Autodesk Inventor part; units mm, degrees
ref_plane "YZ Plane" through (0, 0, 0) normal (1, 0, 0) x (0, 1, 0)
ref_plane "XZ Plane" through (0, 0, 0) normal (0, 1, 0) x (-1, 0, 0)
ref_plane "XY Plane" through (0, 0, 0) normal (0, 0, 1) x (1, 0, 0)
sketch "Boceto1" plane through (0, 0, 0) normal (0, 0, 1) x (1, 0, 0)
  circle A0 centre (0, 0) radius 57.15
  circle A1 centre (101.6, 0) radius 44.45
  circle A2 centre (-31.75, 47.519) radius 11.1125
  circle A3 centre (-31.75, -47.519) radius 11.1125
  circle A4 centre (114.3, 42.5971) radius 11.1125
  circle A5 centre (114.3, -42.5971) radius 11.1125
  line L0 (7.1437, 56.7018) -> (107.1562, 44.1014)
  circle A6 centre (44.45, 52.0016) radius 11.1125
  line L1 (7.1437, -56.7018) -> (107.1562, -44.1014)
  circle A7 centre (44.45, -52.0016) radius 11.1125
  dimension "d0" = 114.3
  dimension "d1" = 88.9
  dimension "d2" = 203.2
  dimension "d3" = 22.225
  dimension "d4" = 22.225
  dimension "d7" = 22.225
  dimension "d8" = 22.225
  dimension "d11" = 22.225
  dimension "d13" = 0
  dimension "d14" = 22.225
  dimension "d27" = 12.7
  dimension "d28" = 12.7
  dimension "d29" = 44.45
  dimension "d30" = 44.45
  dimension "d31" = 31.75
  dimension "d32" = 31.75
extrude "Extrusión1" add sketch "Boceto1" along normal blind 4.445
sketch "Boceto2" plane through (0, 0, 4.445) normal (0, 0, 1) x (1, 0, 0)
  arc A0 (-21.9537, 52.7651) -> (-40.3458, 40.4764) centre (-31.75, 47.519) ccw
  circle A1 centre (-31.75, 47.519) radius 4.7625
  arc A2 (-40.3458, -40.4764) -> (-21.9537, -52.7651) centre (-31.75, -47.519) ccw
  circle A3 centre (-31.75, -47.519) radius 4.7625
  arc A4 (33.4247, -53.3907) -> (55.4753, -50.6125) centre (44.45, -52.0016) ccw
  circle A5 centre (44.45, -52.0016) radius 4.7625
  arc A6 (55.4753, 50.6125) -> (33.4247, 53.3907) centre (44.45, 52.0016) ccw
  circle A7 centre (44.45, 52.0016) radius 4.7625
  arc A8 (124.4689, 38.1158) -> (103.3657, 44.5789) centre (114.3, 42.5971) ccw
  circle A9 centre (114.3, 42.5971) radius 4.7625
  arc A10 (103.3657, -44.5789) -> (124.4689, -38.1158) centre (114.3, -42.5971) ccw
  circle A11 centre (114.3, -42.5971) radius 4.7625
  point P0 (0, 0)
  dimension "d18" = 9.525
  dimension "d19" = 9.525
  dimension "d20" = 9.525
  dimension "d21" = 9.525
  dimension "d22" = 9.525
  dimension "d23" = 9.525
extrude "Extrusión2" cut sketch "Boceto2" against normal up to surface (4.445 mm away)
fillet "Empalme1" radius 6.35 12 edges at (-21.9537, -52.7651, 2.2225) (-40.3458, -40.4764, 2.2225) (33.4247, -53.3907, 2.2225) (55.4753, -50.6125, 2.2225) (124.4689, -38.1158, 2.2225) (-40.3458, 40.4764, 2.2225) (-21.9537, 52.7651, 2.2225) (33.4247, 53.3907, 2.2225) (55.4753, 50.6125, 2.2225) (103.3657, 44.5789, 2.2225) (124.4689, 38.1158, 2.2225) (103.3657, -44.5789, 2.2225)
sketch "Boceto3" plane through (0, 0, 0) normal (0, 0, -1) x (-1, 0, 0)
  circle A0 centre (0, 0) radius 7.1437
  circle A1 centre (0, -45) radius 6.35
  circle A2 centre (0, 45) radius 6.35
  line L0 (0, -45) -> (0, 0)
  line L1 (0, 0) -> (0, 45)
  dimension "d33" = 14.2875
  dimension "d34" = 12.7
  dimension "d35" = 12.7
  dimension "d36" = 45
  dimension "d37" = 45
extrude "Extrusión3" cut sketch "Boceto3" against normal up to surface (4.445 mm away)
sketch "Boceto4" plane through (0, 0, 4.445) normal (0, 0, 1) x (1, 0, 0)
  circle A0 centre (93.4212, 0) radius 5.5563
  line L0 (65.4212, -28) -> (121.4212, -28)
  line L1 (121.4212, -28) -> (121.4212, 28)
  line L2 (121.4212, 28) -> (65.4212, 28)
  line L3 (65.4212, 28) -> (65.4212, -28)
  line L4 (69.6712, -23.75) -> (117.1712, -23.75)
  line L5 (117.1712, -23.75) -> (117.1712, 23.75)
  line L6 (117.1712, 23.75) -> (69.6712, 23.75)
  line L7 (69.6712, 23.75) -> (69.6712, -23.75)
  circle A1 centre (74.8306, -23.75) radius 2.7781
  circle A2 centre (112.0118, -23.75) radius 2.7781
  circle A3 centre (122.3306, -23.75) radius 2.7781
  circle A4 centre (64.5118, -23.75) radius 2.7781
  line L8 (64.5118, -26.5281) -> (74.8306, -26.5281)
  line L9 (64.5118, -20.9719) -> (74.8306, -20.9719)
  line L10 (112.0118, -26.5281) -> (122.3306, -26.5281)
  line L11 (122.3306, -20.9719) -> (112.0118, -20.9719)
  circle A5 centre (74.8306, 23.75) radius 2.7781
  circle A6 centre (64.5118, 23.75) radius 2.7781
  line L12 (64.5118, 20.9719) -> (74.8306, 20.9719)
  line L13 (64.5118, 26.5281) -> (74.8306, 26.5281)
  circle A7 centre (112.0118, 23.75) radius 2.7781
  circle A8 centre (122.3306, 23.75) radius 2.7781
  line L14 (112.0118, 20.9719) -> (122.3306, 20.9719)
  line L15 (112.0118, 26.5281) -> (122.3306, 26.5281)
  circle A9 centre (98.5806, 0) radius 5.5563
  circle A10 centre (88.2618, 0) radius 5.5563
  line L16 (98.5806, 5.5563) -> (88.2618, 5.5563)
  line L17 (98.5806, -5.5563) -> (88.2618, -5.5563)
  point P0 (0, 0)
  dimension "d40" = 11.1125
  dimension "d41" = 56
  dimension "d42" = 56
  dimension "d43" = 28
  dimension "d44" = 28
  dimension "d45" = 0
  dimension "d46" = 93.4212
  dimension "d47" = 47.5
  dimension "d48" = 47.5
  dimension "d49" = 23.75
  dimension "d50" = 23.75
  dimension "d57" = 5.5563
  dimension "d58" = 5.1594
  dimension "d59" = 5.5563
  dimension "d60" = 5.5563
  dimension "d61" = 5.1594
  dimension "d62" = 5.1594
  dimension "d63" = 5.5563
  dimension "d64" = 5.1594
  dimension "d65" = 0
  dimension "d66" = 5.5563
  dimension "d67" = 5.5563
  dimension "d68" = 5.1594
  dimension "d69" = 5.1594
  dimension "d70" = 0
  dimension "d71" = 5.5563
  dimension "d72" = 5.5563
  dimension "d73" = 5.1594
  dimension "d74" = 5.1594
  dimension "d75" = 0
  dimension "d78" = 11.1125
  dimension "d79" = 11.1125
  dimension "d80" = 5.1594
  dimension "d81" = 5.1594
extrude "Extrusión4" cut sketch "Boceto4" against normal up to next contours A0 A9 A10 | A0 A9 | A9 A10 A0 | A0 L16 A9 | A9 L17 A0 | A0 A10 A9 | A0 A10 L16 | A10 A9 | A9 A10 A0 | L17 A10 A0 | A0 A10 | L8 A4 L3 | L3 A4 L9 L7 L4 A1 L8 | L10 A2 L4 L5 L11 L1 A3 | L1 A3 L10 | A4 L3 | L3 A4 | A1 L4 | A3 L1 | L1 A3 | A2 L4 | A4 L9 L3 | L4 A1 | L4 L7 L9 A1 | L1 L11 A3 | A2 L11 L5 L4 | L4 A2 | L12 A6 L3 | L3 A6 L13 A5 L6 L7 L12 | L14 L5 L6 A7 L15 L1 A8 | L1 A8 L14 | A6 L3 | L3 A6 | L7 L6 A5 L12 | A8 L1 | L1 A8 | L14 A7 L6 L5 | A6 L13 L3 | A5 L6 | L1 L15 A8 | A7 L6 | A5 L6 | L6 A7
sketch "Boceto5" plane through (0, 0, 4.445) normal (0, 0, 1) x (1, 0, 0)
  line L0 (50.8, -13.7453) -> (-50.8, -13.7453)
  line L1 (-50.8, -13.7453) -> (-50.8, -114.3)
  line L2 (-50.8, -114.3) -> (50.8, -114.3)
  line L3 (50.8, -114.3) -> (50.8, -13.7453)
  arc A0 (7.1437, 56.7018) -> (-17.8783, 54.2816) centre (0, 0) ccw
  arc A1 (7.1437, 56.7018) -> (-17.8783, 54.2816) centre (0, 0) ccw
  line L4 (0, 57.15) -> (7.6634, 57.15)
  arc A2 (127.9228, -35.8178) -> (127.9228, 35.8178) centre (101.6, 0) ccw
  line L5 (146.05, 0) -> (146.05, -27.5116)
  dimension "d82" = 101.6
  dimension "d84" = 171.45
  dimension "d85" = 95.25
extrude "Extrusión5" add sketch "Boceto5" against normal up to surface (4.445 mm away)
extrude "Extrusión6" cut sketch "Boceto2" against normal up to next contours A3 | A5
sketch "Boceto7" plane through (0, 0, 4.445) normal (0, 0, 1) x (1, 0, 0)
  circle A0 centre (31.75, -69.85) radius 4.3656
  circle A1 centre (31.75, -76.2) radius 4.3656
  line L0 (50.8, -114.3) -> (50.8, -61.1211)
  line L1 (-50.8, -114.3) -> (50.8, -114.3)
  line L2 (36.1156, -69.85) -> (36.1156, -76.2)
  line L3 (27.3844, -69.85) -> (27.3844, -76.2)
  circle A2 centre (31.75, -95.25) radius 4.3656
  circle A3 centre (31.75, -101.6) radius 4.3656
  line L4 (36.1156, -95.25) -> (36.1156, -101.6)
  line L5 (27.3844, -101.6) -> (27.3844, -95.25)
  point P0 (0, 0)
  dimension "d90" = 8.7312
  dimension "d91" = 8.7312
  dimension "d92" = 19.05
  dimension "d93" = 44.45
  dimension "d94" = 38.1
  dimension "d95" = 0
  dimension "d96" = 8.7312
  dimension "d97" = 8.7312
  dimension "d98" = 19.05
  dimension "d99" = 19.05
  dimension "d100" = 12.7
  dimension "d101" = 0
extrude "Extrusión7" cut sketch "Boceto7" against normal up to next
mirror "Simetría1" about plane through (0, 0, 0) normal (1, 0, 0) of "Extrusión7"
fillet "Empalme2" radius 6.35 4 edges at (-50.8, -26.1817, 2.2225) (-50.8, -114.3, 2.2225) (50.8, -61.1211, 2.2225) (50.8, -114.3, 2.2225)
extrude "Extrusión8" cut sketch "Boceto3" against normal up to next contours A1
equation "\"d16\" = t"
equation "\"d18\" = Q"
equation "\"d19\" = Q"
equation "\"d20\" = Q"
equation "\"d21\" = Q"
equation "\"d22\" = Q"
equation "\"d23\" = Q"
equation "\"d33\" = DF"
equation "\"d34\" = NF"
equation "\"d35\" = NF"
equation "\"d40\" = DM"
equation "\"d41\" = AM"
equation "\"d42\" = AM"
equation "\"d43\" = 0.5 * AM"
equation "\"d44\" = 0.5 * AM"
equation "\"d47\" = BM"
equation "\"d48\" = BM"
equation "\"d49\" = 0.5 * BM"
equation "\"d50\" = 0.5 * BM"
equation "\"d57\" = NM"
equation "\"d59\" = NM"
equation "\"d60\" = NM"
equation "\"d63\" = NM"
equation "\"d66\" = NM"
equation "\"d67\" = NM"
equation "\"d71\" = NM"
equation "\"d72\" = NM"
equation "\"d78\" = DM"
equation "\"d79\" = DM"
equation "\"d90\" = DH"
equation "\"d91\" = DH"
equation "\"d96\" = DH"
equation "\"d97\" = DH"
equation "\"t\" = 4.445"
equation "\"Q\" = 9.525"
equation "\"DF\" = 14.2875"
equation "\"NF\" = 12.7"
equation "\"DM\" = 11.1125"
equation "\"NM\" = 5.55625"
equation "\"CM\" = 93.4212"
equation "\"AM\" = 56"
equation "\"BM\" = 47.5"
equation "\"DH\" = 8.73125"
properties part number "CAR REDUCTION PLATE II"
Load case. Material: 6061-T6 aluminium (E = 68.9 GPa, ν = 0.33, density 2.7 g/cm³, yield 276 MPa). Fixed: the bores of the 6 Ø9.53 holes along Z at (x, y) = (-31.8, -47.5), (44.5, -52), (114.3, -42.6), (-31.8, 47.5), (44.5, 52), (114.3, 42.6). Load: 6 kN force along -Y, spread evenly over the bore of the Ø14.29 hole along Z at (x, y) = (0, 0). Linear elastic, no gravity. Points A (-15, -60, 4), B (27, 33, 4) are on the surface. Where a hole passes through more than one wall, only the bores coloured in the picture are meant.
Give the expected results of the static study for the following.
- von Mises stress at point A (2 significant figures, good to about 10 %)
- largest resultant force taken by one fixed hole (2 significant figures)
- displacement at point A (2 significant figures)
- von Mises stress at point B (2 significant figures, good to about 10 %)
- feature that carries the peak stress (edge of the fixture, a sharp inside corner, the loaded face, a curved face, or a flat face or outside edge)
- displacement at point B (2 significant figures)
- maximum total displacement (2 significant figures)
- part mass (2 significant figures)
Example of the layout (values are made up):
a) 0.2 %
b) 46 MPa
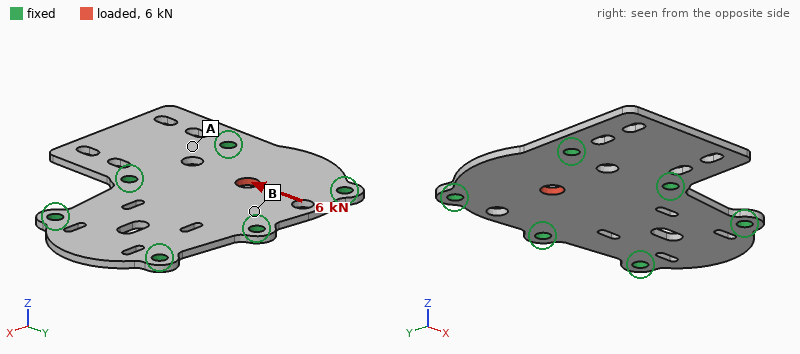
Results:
a) 4.7 MPa
b) 1.9 kN
c) 2.9 µm
d) 11 MPa
e) the loaded face
f) 4.7 µm
g) 14 µm
h) 290 g
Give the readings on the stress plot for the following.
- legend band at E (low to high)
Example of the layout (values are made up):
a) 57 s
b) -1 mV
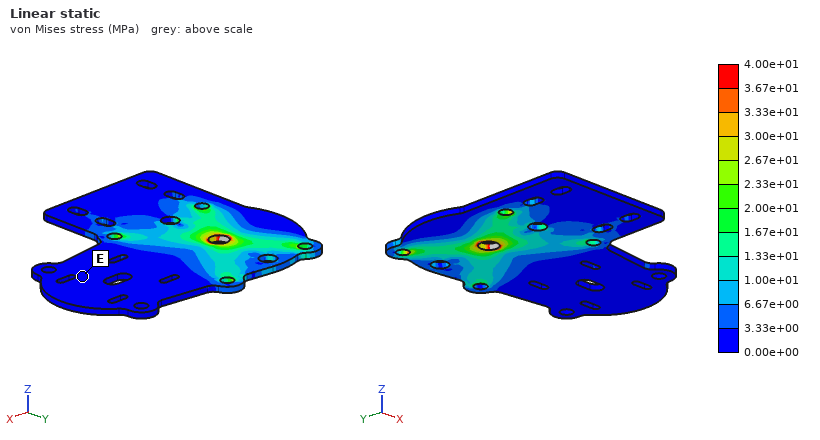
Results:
a) 0.00e+00 to 3.33e+00 MPa
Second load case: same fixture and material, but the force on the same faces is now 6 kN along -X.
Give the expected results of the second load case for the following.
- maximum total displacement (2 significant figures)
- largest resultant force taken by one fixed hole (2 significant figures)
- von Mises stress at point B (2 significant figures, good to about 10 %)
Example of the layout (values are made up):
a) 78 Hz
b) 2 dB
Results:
a) 17 µm
b) 1.5 kN
c) 10 MPa
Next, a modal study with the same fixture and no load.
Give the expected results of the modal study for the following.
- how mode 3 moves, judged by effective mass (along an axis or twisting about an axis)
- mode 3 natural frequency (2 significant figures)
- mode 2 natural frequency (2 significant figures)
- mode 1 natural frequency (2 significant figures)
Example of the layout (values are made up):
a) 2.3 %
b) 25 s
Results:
a) along Z
b) 2100 Hz
c) 1600 Hz
d) 840 Hz
